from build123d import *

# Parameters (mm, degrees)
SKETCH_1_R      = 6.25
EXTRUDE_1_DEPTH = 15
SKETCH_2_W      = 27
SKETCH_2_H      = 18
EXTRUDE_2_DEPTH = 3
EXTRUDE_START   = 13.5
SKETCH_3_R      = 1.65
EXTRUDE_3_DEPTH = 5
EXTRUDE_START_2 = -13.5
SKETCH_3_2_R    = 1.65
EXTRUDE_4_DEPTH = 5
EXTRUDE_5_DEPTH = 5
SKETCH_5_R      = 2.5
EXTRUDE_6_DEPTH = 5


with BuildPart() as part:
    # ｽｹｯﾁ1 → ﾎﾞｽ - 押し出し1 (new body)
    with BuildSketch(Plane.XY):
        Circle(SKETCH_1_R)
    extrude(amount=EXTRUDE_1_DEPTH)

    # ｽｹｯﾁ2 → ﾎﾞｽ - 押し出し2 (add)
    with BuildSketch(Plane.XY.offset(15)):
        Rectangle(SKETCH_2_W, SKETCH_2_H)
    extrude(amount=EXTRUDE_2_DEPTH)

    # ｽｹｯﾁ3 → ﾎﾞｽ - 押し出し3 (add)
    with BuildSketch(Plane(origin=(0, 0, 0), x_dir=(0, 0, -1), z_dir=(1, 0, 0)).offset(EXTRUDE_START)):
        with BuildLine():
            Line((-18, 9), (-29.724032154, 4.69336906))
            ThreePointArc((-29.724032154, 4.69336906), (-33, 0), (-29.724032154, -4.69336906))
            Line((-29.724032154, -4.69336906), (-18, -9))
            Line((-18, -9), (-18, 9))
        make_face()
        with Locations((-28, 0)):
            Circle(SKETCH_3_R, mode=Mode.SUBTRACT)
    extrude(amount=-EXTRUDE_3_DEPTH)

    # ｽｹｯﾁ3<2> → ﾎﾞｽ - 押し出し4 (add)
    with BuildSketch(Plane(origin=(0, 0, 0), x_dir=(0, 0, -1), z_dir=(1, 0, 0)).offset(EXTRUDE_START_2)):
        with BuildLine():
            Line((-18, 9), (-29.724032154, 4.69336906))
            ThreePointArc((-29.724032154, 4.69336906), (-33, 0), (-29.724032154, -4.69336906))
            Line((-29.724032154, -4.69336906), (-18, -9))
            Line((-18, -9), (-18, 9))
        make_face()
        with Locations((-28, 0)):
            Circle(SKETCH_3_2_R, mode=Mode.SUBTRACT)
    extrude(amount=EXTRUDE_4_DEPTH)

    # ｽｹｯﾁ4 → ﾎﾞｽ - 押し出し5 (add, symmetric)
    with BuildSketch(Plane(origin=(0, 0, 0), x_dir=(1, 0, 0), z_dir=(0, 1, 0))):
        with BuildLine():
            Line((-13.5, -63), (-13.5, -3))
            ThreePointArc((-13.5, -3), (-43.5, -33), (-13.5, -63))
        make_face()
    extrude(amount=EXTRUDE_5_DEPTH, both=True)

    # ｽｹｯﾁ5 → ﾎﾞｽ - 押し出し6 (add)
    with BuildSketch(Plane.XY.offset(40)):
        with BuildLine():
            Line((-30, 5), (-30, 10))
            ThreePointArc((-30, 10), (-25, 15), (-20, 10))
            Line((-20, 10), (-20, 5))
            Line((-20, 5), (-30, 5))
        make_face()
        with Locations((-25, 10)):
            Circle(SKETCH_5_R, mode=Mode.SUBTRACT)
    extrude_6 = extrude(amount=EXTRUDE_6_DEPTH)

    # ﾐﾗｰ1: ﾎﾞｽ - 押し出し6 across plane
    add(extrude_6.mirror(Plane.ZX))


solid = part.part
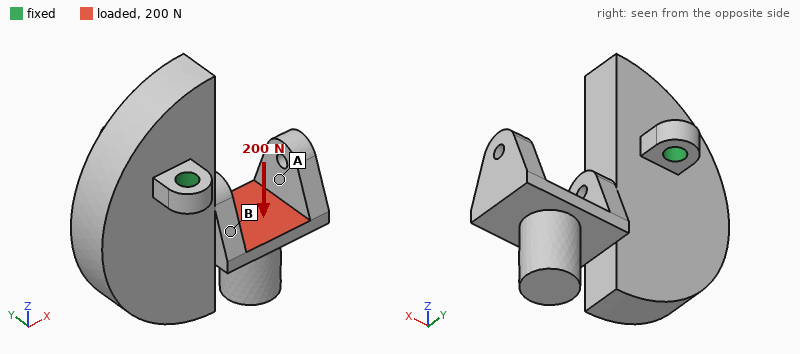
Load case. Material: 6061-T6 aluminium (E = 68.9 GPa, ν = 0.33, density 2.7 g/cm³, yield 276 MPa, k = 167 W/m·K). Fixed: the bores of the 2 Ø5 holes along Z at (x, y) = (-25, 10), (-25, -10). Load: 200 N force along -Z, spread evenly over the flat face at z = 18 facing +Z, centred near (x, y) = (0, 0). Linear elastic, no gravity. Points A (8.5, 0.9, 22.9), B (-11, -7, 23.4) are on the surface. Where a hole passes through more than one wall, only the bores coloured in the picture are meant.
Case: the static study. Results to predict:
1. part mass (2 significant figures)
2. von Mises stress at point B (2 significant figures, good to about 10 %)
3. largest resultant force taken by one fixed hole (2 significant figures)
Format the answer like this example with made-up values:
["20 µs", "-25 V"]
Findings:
["54 g", "9.3 MPa", "100 N"]
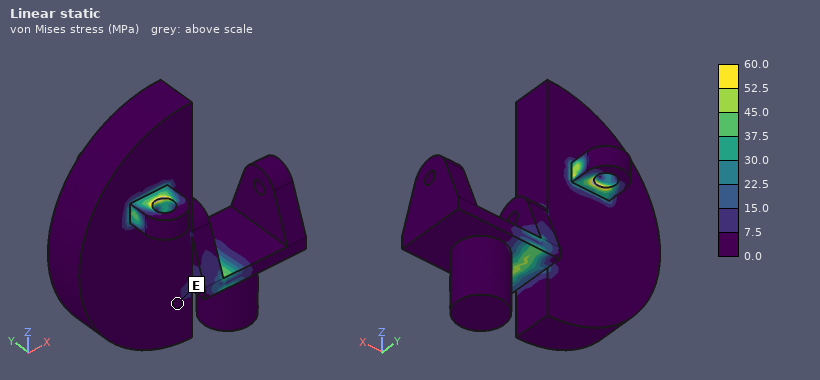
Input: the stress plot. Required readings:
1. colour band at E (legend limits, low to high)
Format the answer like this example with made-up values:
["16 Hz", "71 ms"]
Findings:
["0.0 to 7.5 MPa"]
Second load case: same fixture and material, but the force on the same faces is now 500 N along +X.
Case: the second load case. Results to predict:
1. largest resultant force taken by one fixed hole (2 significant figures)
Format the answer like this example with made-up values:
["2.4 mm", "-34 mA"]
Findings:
["250 N"]
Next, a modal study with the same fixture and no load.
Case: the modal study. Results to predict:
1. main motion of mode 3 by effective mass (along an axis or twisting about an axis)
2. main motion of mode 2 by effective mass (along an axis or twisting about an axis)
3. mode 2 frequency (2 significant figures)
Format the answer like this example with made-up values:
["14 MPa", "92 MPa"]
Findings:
["along X", "along Y", "2700 Hz"]
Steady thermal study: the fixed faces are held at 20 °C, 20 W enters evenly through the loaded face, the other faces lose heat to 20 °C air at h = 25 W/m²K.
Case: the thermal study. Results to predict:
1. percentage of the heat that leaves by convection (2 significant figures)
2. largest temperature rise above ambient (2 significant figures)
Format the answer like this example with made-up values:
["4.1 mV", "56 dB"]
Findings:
["14 %", "38 K"]
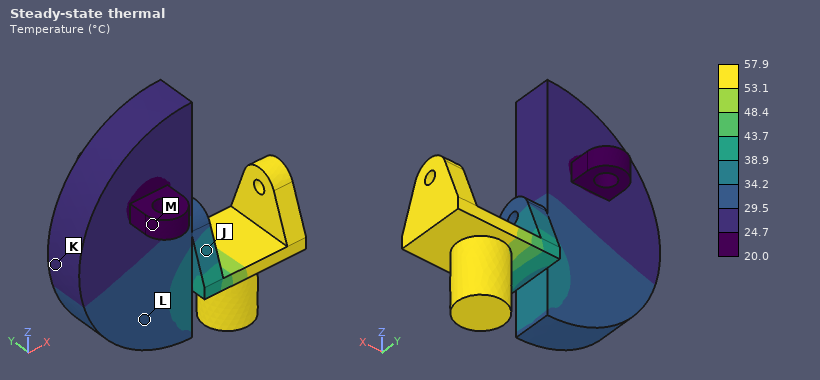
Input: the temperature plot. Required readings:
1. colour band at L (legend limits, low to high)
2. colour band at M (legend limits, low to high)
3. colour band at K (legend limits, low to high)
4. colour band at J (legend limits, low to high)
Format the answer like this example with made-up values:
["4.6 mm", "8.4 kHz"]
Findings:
["29.5 to 34.2 °C", "20.0 to 24.7 °C", "24.7 to 29.5 °C", "34.2 to 38.9 °C"]
